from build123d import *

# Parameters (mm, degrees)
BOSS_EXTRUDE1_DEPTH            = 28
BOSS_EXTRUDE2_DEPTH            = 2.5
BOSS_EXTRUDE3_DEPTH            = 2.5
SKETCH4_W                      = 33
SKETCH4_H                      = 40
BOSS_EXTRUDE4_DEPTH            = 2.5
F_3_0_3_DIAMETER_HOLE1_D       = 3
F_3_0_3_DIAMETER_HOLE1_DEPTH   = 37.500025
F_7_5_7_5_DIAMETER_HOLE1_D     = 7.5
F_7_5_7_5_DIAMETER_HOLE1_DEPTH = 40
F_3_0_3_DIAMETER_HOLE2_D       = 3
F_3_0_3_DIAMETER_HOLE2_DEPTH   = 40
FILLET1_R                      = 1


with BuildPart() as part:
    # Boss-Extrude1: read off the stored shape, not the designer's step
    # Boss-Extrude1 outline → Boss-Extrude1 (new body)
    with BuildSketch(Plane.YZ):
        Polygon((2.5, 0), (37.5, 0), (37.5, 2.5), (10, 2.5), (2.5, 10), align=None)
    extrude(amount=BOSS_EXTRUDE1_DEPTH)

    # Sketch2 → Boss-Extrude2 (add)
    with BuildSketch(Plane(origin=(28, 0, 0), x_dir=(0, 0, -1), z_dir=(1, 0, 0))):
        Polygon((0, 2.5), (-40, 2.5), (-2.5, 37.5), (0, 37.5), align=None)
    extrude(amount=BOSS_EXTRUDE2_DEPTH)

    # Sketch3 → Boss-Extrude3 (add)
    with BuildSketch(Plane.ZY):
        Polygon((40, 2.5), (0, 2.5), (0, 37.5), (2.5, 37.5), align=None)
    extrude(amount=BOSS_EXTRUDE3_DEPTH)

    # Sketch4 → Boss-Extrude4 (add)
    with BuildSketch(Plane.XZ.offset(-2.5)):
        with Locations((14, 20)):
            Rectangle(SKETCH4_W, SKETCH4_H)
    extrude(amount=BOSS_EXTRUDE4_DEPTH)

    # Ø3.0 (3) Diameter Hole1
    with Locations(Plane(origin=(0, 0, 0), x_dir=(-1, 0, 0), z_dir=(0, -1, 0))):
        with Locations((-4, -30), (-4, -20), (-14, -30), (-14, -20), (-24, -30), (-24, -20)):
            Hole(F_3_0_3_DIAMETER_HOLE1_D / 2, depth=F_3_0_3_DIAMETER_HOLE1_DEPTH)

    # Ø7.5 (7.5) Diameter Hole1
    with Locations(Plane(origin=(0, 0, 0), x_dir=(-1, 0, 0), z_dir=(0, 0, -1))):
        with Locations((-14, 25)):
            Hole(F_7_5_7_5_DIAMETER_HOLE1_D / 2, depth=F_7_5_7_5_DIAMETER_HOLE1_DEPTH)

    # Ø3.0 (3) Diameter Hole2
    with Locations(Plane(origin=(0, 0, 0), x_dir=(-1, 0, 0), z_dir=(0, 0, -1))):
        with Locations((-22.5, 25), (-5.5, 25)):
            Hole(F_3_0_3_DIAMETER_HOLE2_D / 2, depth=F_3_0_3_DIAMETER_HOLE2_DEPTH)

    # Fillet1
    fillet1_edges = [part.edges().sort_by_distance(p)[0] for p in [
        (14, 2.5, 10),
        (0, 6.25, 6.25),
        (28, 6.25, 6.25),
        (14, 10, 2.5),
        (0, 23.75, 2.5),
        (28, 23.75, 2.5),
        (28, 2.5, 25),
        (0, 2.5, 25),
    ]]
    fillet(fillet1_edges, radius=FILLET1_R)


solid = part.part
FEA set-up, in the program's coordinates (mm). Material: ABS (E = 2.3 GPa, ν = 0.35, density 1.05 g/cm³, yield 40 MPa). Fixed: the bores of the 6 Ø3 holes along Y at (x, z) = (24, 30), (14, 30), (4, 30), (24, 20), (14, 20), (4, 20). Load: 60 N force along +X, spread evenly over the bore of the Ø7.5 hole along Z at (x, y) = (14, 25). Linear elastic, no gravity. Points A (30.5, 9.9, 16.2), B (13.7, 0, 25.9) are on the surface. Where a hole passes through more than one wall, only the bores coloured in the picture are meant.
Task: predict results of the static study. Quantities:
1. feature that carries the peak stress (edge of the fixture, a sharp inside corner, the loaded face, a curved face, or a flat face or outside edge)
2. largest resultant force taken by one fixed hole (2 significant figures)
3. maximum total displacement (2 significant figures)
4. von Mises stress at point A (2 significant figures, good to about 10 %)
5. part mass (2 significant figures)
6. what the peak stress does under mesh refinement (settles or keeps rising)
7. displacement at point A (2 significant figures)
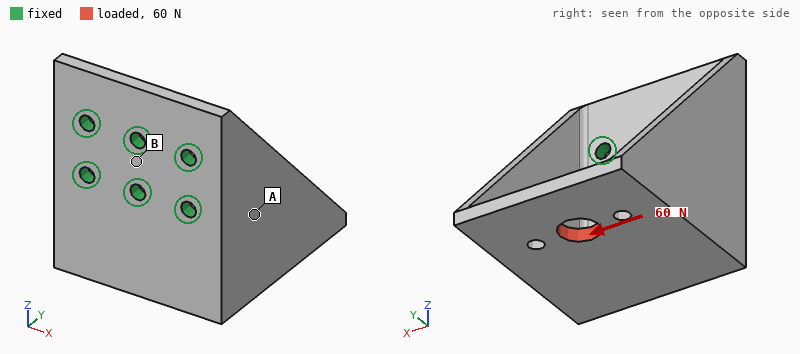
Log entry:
edge of the fixture
88 N
0.59 mm
2.8 MPa
11 g
keeps rising
0.16 mm
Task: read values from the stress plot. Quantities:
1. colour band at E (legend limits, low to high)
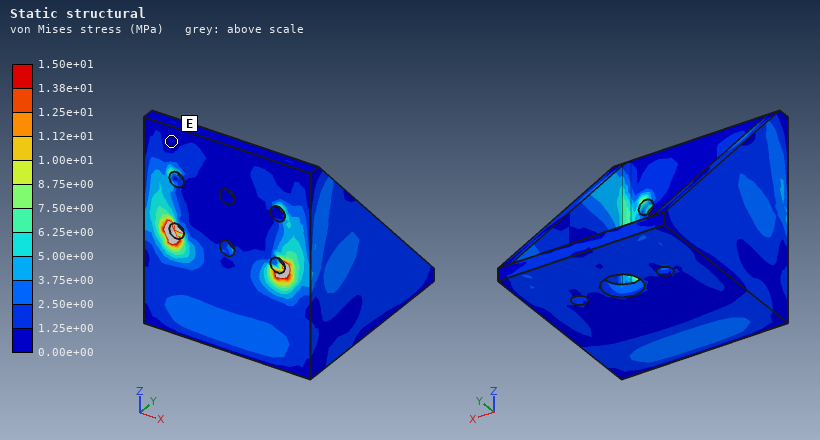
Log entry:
0.00e+00 to 1.25e+00 MPa
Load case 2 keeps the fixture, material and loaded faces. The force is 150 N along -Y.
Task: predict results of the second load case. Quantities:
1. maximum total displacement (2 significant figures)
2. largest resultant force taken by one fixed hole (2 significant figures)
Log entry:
0.73 mm
150 N
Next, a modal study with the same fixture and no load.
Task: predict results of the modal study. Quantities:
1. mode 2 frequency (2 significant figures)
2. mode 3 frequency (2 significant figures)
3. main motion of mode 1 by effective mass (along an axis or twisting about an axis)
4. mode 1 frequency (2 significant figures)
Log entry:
1000 Hz
2200 Hz
along X
910 Hz
